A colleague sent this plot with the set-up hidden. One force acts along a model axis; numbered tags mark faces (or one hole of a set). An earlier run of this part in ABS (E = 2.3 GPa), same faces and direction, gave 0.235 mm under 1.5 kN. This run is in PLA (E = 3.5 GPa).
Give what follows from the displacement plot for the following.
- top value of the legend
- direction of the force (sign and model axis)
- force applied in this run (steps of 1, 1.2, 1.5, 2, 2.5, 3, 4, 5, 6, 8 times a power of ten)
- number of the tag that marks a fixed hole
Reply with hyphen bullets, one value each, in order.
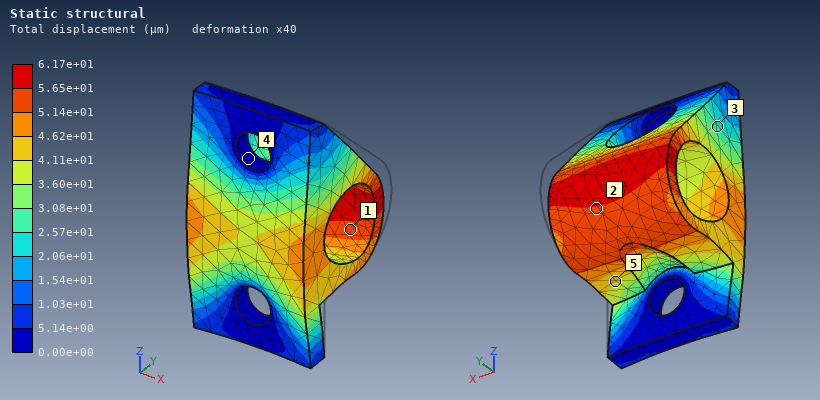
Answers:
- 6.17e+01 µm
- -Y
- 600 N
- 4
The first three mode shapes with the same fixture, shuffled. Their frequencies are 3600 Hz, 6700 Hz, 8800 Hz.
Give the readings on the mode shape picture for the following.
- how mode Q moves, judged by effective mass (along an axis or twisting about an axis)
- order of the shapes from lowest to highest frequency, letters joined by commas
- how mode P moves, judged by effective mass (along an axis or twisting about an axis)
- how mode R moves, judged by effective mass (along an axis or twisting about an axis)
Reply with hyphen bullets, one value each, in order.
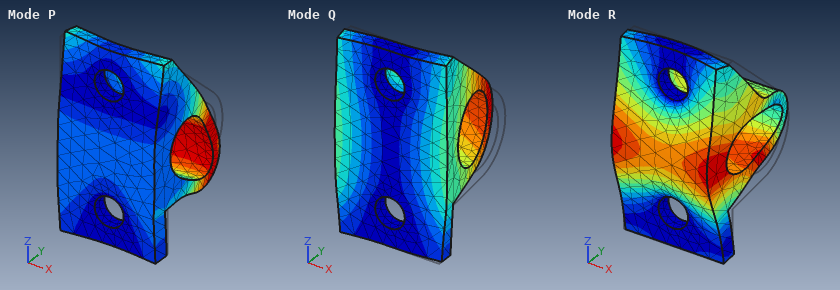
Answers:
- along X
- Q, P, R
- along Z
- along Y
